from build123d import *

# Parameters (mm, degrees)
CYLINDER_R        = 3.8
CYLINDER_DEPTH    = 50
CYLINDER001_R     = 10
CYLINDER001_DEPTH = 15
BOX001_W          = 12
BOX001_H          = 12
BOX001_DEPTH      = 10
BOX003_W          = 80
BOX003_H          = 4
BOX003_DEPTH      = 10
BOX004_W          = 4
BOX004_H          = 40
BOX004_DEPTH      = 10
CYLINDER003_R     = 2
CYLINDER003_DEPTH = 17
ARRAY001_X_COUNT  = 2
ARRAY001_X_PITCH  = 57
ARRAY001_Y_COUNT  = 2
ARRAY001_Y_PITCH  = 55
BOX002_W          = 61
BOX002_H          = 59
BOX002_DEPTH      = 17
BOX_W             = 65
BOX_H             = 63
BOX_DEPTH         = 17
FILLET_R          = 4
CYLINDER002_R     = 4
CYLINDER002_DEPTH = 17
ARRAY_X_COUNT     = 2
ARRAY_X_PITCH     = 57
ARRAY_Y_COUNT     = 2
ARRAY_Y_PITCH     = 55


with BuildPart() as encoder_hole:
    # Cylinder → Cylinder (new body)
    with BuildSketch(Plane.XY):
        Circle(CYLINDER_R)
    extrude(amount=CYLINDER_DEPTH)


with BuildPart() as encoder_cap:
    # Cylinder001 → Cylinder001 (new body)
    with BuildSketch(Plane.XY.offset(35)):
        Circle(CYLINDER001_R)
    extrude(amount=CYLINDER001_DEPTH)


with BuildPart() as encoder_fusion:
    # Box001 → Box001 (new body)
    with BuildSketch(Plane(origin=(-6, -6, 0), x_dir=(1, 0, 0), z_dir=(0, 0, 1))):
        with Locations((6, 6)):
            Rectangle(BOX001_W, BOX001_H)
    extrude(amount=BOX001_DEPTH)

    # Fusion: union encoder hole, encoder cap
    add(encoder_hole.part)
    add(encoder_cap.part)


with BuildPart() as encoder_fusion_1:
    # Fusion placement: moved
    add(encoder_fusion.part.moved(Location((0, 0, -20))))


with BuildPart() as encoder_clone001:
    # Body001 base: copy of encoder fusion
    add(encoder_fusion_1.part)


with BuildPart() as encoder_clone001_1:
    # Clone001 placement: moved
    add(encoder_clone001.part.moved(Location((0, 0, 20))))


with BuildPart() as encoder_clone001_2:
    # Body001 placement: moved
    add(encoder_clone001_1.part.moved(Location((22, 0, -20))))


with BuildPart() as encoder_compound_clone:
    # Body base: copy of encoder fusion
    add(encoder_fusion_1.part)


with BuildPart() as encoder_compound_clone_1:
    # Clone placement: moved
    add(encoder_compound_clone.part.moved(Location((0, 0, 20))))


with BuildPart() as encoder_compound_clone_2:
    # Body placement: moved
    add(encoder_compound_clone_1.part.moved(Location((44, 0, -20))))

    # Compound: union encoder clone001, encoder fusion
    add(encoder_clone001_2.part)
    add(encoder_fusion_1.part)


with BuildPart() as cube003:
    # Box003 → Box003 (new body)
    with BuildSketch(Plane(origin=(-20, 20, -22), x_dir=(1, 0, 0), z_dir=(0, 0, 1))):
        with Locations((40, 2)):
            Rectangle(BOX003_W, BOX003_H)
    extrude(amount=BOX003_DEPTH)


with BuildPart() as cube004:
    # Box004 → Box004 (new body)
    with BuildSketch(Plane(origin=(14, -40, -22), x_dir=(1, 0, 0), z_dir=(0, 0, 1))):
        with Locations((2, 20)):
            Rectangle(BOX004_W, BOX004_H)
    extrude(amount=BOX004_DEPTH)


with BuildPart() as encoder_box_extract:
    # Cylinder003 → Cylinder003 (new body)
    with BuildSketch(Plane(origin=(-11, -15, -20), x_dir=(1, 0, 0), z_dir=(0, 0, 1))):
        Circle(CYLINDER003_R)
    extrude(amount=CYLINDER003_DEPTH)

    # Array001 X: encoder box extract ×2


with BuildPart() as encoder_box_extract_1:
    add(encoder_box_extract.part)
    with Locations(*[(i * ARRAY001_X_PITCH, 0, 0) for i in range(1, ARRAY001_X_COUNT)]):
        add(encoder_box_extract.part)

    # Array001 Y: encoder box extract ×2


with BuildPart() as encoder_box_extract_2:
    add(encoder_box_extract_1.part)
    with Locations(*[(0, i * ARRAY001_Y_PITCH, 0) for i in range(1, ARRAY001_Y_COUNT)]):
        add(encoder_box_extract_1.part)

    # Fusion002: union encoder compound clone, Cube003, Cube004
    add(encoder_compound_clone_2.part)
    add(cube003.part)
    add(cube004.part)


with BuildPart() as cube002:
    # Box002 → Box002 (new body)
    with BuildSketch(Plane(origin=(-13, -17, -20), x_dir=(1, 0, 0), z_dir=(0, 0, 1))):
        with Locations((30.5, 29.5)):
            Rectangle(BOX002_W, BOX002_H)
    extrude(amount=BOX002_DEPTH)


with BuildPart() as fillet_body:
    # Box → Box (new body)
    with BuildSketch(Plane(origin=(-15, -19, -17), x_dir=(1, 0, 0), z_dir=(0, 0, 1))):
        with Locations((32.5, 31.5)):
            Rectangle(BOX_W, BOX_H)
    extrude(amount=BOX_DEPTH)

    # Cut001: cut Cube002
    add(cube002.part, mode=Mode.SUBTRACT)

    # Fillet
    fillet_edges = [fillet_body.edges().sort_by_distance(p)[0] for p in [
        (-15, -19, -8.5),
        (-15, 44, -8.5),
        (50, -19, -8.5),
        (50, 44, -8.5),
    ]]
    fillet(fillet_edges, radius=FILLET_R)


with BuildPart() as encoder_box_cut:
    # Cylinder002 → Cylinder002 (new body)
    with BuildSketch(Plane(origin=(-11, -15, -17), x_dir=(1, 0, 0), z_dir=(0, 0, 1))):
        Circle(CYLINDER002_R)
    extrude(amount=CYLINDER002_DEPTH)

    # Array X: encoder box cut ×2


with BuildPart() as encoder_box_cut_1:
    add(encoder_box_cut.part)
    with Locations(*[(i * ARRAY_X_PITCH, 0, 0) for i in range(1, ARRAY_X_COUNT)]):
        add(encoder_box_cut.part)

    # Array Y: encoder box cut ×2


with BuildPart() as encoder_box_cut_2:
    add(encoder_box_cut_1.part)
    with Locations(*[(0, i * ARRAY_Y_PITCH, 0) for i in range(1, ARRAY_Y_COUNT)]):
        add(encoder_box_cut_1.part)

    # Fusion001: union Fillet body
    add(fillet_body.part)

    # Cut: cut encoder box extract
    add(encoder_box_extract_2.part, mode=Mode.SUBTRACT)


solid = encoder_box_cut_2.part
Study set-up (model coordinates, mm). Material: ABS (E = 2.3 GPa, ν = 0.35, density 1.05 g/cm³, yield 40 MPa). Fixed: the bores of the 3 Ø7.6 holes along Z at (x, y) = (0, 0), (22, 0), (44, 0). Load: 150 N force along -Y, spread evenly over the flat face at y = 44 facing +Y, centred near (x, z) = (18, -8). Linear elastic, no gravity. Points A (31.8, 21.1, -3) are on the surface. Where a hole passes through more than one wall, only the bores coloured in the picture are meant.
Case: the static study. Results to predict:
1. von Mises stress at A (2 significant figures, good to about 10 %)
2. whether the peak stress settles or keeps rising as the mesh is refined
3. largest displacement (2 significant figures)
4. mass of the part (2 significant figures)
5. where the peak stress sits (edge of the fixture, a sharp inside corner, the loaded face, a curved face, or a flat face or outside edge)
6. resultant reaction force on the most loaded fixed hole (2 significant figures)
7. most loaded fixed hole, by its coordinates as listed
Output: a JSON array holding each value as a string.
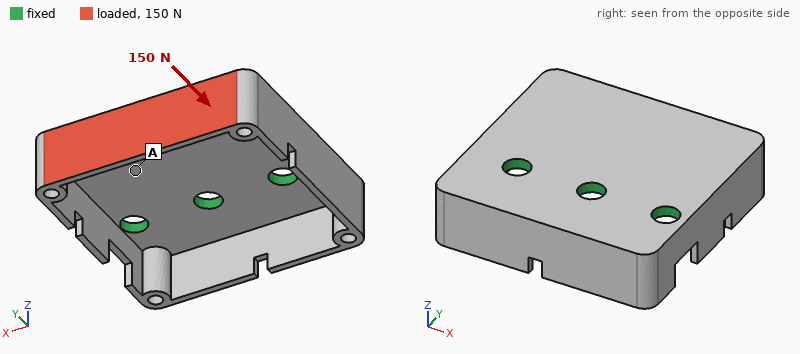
["2.4 MPa", "keeps rising", "1.1 mm", "20 g", "edge of the fixture", "83 N", "(0, 0)"]
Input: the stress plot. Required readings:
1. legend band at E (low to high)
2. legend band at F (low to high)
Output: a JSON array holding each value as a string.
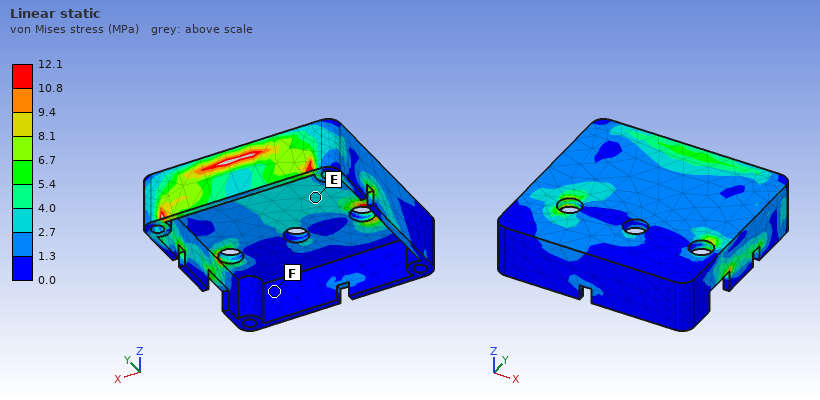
["2.7 to 4.0 MPa", "0.0 to 1.3 MPa"]
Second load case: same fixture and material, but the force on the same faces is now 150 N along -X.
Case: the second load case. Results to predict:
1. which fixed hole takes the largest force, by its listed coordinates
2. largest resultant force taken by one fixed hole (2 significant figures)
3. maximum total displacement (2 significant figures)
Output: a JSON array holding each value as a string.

["(0, 0)", "160 N", "0.90 mm"]
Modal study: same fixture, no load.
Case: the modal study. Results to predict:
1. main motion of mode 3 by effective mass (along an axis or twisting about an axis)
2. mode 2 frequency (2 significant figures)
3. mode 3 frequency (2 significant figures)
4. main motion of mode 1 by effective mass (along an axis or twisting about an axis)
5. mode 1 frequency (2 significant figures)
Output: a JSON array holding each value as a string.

["along Z", "670 Hz", "1700 Hz", "along Z", "460 Hz"]
